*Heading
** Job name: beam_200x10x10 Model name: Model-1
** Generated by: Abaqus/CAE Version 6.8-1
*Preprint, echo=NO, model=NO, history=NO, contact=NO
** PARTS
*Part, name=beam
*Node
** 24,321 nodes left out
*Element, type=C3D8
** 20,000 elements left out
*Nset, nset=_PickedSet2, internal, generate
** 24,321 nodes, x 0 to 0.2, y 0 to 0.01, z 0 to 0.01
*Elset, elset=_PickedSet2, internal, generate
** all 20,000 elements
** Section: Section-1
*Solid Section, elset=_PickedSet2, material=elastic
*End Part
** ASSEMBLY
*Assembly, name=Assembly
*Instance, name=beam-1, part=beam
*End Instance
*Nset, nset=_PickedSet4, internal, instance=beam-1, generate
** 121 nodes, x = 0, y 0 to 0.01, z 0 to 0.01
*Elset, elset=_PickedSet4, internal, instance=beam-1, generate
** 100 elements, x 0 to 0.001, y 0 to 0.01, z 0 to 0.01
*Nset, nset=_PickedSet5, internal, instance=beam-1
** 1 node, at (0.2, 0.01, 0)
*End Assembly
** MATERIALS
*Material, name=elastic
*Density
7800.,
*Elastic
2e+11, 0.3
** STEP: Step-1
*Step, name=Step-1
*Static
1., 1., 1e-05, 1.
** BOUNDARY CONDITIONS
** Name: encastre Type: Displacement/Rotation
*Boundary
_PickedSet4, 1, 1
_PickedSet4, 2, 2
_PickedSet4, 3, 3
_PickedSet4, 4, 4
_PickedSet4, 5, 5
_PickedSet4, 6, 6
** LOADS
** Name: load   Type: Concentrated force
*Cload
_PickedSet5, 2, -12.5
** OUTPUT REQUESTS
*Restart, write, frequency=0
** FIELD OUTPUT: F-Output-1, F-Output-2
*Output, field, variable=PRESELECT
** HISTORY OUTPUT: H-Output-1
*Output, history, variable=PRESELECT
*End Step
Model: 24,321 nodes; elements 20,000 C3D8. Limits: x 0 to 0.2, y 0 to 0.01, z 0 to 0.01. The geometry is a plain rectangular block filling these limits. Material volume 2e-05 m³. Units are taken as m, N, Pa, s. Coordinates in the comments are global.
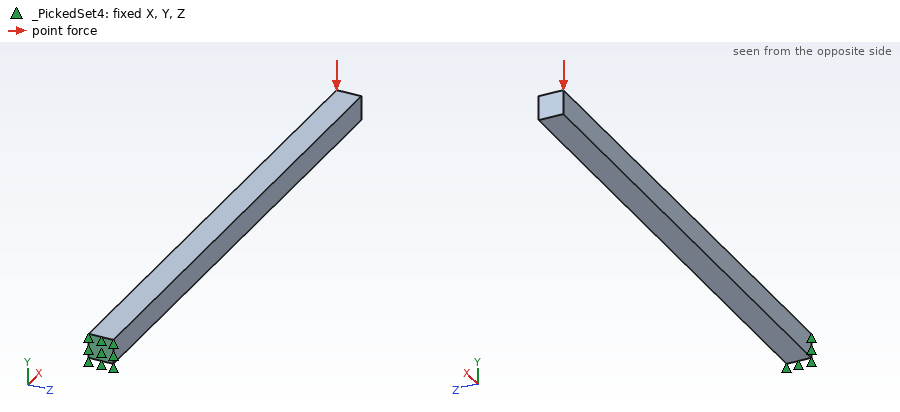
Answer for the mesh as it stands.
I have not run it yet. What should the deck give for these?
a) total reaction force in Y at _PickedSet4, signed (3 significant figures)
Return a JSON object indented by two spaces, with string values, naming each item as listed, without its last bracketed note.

{
  "total reaction force in Y at _PickedSet4, signed": "12.5 N"
}
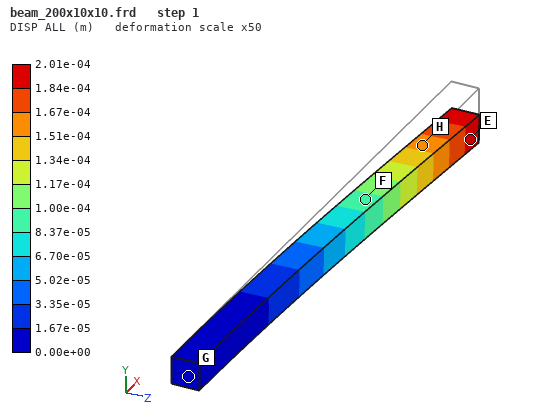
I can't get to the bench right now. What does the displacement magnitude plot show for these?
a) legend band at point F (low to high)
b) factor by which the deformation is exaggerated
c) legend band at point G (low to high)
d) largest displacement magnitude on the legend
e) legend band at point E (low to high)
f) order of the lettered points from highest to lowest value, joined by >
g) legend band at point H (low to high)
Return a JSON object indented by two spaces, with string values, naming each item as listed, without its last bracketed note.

{
  "legend band at point F": "8.37e-05 to 1.00e-04 m",
  "factor by which the deformation is exaggerated": "50",
  "legend band at point G": "0.00e+00 to 1.67e-05 m",
  "largest displacement magnitude on the legend": "2.01e-04 m",
  "legend band at point E": "1.84e-04 to 2.01e-04 m",
  "order of the lettered points from highest to lowest value, joined by >": "E > H > F > G",
  "legend band at point H": "1.51e-04 to 1.67e-04 m"
}
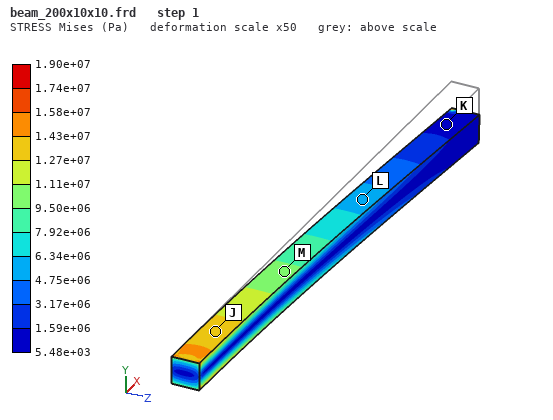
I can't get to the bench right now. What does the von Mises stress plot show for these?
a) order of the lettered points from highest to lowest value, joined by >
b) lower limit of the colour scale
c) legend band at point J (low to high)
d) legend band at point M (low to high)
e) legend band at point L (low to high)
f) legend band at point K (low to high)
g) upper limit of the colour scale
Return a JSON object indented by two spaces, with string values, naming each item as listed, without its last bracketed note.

{
  "order of the lettered points from highest to lowest value, joined by >": "J > M > L > K",
  "lower limit of the colour scale": "5.48e+03 Pa",
  "legend band at point J": "1.27e+07 to 1.43e+07 Pa",
  "legend band at point M": "9.50e+06 to 1.11e+07 Pa",
  "legend band at point L": "4.75e+06 to 6.34e+06 Pa",
  "legend band at point K": "5.48e+03 to 1.59e+06 Pa",
  "upper limit of the colour scale": "1.90e+07 Pa"
}
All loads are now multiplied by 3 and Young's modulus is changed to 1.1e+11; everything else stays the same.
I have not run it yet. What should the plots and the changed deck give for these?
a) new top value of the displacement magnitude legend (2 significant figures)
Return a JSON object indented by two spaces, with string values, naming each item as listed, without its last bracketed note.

{
  "new top value of the displacement magnitude legend": "0.0011 m"
}
